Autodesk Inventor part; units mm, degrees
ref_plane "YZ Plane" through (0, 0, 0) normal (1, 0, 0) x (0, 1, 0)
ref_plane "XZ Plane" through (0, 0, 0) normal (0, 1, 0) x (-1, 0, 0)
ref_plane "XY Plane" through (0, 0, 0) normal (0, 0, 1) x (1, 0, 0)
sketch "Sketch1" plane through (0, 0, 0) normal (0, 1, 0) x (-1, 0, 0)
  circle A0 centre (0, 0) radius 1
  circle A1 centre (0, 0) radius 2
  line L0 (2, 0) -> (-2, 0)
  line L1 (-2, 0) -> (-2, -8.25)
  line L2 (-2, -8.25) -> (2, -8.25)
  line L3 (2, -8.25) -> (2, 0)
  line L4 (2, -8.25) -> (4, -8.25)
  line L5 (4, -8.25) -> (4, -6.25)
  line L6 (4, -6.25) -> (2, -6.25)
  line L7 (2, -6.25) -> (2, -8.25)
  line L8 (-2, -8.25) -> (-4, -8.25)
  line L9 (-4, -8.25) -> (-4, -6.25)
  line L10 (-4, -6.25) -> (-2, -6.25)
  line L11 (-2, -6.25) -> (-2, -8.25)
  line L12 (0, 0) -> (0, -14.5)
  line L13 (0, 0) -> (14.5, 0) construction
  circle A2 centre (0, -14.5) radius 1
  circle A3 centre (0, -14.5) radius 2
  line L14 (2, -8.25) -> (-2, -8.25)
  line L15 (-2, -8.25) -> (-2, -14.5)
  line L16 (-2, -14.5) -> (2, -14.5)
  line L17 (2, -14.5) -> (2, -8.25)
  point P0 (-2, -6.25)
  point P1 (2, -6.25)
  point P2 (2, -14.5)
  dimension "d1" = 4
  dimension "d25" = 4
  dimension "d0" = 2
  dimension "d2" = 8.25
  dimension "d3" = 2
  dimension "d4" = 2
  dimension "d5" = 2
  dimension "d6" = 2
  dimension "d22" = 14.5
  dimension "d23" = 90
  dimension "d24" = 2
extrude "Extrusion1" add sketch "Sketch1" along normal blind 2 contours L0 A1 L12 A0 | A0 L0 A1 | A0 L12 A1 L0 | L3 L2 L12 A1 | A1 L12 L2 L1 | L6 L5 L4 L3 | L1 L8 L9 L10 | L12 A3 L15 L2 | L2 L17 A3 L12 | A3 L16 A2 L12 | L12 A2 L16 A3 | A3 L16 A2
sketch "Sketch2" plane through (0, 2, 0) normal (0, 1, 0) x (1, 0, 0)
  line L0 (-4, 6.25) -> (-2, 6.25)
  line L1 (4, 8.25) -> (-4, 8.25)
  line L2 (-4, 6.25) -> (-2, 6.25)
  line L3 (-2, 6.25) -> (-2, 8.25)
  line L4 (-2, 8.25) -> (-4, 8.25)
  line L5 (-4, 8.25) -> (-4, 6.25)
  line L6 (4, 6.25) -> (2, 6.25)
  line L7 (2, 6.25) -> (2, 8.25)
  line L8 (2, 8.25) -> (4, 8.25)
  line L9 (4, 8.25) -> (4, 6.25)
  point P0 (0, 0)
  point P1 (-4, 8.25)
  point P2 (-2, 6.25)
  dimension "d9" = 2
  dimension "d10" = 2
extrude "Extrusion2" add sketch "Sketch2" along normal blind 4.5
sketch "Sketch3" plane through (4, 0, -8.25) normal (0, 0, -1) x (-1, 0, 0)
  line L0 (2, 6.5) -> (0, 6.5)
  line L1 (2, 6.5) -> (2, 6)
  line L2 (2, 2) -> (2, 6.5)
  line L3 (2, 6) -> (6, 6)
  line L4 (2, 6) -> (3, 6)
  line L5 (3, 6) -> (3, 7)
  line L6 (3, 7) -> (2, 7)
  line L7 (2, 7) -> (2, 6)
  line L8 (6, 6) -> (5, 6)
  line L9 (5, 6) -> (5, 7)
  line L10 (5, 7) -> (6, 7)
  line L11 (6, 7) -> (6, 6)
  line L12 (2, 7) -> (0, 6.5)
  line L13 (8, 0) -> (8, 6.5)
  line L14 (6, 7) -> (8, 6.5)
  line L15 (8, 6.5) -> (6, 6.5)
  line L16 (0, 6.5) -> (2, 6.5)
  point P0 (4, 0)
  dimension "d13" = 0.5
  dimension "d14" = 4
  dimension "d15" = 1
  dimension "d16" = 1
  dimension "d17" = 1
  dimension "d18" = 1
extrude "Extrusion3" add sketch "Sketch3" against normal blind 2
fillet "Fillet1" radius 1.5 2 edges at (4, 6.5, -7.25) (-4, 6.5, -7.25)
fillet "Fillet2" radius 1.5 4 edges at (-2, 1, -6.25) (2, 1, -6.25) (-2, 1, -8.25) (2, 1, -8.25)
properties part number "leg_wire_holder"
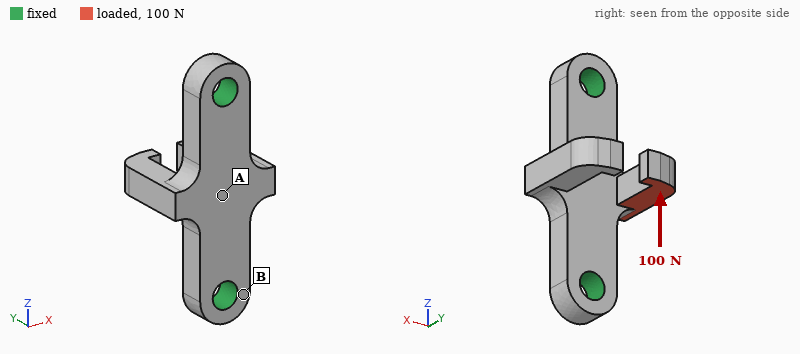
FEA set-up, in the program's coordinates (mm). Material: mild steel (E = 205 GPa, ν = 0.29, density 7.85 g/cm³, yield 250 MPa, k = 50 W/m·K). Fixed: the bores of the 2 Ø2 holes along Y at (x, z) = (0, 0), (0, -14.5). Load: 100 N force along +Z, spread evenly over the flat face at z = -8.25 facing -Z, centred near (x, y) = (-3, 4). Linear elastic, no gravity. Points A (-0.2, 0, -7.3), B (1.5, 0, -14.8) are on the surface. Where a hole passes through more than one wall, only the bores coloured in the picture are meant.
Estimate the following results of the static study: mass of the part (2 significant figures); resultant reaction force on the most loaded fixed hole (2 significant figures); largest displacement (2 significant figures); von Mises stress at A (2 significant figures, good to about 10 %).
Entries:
1.5 g
66 N
17 µm
41 MPa
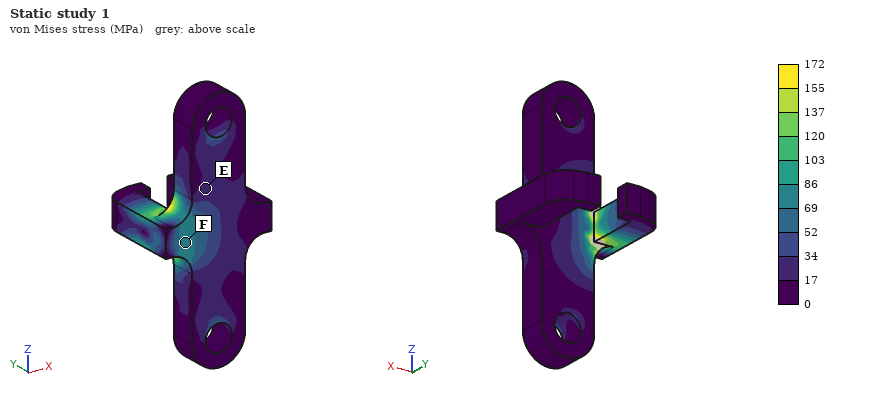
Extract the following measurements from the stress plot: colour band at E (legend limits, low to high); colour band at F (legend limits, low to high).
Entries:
17 to 34 MPa
69 to 86 MPa
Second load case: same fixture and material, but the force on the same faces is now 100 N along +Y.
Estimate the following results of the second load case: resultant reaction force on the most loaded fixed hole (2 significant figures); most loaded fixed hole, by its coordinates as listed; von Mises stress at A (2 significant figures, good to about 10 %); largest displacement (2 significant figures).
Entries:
61 N
(0, -14.5)
60 MPa
15 µm
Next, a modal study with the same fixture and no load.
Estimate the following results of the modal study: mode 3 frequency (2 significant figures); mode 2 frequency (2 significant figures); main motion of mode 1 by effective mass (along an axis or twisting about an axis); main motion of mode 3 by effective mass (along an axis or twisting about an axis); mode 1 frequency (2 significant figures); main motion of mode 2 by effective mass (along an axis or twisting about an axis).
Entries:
34 kHz
29 kHz
along X
along Z
21 kHz
along Y
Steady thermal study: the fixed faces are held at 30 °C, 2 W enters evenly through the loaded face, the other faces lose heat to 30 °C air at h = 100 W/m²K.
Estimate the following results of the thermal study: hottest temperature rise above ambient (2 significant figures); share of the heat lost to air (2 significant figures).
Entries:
50 K
17 %
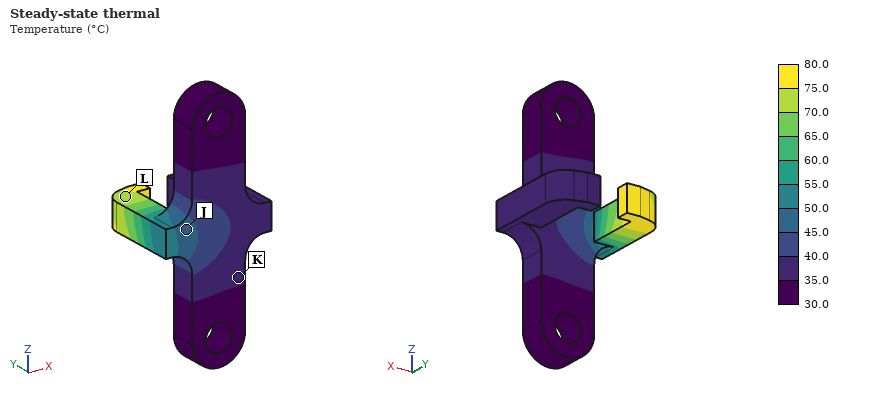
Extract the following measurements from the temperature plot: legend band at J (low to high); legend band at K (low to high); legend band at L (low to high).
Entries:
45.0 to 50.0 °C
35.0 to 40.0 °C
70.0 to 75.0 °C
